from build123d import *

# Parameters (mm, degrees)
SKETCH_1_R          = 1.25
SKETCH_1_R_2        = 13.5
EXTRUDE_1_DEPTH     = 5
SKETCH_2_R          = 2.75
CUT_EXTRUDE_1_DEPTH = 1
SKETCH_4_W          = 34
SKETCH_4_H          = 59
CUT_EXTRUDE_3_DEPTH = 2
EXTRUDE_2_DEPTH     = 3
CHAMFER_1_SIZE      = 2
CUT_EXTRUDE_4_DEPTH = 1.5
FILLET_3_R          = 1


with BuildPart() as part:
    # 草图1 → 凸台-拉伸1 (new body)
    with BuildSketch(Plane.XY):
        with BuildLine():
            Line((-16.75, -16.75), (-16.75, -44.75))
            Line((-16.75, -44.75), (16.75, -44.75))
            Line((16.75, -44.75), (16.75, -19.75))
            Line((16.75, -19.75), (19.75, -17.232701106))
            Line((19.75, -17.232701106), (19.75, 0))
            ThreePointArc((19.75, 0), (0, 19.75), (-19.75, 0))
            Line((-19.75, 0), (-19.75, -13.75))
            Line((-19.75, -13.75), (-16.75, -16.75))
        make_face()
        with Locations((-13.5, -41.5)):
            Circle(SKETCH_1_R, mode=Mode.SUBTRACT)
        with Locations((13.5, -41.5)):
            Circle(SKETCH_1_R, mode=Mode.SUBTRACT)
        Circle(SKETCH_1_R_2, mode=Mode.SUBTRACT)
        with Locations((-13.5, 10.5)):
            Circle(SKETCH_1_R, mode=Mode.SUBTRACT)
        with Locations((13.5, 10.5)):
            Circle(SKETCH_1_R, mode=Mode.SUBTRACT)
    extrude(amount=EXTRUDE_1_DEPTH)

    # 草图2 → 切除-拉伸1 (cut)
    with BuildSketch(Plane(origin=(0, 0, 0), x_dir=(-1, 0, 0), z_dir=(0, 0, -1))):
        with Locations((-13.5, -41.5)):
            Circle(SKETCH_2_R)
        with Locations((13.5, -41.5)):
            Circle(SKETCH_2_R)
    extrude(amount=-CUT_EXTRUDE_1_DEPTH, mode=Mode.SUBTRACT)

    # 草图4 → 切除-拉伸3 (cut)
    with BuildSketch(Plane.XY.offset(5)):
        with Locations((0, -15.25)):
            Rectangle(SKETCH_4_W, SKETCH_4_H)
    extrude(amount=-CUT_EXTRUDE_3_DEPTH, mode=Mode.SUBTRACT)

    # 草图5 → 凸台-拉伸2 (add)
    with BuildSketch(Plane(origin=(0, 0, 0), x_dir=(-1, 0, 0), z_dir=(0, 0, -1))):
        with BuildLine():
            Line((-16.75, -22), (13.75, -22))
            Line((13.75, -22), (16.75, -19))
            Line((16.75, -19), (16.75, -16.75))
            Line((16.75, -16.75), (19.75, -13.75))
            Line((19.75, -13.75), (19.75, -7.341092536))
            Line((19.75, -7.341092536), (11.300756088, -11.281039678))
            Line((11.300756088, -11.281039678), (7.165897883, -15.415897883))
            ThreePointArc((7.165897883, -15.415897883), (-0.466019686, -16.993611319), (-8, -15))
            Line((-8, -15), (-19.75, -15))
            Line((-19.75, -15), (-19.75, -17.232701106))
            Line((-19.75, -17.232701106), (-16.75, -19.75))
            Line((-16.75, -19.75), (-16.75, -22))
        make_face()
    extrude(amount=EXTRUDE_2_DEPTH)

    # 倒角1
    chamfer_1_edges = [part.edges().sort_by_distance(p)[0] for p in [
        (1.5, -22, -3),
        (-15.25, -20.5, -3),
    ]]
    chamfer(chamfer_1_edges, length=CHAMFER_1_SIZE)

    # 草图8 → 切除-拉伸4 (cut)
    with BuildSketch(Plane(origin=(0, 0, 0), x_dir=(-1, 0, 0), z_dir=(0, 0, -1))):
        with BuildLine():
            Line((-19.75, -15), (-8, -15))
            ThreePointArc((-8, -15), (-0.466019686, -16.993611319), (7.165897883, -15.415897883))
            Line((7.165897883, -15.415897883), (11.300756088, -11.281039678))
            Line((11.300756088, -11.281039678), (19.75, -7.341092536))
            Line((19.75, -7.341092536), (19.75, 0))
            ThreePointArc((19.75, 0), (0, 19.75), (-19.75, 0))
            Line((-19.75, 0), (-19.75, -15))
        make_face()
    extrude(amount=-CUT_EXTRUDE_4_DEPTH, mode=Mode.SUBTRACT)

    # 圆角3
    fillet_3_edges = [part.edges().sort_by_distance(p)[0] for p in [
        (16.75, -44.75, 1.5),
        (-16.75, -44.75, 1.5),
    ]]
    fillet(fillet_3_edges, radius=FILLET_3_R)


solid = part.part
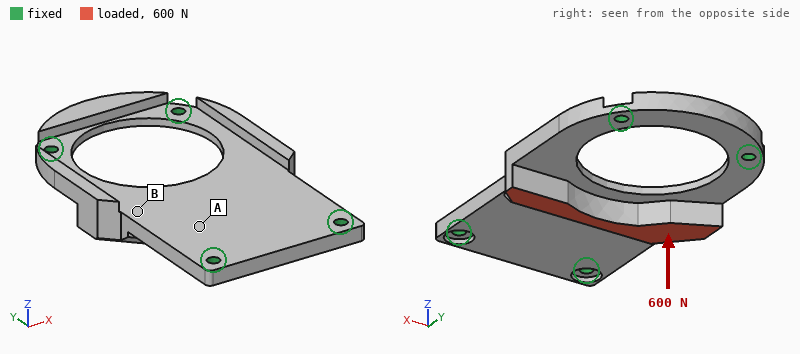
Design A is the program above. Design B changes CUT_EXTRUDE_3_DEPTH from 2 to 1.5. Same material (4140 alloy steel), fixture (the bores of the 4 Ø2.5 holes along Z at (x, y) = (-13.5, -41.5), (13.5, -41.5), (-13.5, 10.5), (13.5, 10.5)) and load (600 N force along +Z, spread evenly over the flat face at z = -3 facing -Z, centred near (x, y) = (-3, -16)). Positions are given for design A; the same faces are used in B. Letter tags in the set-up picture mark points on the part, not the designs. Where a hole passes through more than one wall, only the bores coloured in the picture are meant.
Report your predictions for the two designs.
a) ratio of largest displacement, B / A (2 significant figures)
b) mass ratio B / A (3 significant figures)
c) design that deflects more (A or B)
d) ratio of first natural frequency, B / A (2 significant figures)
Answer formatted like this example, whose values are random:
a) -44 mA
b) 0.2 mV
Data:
a) 0.71
b) 1.13
c) A
d) 1.1
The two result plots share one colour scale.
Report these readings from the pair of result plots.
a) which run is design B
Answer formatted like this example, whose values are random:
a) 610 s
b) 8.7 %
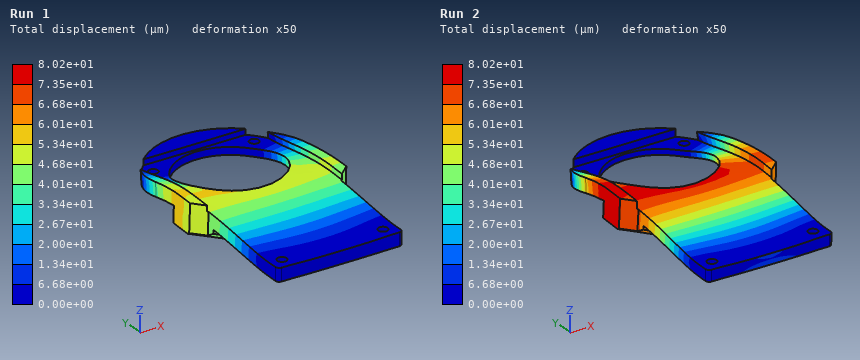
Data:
a) Run 1
